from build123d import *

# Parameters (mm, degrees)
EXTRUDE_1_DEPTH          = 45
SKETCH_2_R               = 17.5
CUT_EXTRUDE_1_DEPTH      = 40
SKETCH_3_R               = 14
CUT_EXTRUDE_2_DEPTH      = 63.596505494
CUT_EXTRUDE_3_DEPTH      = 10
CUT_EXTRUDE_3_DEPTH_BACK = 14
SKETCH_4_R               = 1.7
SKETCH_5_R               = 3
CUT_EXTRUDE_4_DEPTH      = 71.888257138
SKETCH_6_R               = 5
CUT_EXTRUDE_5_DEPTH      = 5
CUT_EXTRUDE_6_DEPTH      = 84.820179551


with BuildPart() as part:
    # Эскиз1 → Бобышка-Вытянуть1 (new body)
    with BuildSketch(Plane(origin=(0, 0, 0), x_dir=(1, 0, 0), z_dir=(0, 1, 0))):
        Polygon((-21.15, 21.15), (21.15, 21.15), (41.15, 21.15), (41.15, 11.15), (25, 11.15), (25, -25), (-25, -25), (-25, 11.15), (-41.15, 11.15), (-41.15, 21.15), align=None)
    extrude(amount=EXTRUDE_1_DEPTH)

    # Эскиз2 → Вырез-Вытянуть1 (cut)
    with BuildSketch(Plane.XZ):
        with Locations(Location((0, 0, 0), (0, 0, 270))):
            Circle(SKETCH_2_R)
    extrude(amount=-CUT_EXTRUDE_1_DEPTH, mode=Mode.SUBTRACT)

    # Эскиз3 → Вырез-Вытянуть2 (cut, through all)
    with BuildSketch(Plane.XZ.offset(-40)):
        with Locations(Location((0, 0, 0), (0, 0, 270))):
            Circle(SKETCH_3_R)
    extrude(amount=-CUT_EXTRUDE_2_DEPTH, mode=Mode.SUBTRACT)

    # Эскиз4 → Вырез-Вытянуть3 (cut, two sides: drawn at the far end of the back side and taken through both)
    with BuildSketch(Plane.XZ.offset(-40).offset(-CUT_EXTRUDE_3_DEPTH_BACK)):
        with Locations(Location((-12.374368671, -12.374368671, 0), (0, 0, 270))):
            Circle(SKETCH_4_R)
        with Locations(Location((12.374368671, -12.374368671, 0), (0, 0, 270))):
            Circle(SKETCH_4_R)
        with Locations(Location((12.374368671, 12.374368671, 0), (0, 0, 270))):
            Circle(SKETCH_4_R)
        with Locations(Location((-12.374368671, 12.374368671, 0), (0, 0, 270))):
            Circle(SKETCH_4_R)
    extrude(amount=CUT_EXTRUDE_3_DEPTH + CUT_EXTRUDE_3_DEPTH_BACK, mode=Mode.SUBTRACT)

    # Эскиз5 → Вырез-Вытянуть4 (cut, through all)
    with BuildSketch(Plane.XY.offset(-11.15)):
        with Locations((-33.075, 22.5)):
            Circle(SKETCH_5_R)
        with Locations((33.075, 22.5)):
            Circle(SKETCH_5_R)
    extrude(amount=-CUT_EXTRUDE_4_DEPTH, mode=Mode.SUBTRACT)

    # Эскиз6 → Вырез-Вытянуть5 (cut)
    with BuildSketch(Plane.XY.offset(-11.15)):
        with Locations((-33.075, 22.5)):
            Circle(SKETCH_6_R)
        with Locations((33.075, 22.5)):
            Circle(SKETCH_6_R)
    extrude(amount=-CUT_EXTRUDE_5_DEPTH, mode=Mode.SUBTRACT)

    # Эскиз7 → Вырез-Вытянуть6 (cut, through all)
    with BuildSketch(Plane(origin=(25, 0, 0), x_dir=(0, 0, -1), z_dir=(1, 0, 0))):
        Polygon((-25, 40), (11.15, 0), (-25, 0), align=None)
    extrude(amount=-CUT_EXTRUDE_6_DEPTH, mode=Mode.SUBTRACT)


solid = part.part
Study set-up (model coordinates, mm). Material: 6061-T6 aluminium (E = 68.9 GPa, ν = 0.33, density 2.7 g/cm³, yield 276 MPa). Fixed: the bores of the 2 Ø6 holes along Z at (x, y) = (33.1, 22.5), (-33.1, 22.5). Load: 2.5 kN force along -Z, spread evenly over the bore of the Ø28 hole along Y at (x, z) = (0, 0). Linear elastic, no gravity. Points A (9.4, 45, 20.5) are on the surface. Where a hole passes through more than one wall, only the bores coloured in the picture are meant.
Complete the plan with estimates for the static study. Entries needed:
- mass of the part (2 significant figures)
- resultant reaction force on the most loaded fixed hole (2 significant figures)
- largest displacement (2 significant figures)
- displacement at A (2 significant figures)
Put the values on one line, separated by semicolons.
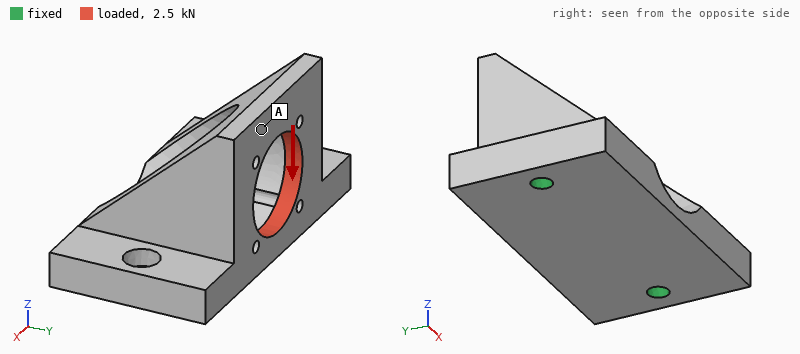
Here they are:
140 g; 1.3 kN; 0.16 mm; 0.15 mm
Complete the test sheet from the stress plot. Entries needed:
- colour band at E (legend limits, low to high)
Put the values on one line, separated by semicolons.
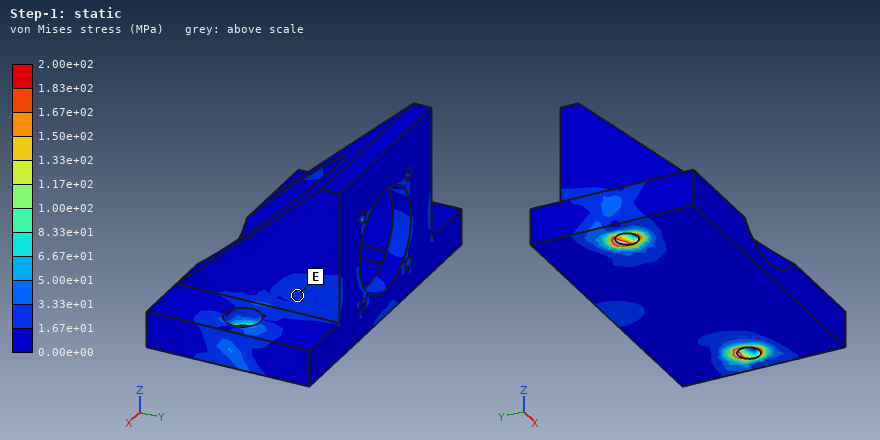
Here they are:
1.67e+01 to 3.33e+01 MPa
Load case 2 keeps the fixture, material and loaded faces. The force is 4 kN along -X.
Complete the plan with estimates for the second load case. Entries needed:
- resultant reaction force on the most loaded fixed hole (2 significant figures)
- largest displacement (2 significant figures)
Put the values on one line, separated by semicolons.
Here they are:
2.6 kN; 39 µm
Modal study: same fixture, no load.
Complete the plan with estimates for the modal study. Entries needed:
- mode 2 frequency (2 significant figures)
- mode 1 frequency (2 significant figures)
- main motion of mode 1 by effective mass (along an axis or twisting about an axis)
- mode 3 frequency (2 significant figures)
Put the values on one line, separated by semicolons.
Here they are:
6300 Hz; 2500 Hz; along Y; 6500 Hz
